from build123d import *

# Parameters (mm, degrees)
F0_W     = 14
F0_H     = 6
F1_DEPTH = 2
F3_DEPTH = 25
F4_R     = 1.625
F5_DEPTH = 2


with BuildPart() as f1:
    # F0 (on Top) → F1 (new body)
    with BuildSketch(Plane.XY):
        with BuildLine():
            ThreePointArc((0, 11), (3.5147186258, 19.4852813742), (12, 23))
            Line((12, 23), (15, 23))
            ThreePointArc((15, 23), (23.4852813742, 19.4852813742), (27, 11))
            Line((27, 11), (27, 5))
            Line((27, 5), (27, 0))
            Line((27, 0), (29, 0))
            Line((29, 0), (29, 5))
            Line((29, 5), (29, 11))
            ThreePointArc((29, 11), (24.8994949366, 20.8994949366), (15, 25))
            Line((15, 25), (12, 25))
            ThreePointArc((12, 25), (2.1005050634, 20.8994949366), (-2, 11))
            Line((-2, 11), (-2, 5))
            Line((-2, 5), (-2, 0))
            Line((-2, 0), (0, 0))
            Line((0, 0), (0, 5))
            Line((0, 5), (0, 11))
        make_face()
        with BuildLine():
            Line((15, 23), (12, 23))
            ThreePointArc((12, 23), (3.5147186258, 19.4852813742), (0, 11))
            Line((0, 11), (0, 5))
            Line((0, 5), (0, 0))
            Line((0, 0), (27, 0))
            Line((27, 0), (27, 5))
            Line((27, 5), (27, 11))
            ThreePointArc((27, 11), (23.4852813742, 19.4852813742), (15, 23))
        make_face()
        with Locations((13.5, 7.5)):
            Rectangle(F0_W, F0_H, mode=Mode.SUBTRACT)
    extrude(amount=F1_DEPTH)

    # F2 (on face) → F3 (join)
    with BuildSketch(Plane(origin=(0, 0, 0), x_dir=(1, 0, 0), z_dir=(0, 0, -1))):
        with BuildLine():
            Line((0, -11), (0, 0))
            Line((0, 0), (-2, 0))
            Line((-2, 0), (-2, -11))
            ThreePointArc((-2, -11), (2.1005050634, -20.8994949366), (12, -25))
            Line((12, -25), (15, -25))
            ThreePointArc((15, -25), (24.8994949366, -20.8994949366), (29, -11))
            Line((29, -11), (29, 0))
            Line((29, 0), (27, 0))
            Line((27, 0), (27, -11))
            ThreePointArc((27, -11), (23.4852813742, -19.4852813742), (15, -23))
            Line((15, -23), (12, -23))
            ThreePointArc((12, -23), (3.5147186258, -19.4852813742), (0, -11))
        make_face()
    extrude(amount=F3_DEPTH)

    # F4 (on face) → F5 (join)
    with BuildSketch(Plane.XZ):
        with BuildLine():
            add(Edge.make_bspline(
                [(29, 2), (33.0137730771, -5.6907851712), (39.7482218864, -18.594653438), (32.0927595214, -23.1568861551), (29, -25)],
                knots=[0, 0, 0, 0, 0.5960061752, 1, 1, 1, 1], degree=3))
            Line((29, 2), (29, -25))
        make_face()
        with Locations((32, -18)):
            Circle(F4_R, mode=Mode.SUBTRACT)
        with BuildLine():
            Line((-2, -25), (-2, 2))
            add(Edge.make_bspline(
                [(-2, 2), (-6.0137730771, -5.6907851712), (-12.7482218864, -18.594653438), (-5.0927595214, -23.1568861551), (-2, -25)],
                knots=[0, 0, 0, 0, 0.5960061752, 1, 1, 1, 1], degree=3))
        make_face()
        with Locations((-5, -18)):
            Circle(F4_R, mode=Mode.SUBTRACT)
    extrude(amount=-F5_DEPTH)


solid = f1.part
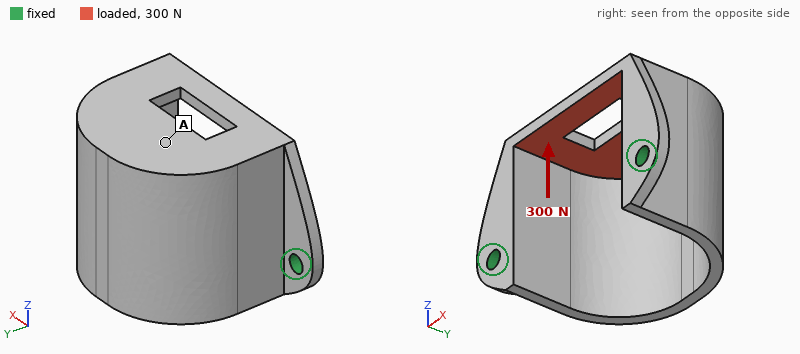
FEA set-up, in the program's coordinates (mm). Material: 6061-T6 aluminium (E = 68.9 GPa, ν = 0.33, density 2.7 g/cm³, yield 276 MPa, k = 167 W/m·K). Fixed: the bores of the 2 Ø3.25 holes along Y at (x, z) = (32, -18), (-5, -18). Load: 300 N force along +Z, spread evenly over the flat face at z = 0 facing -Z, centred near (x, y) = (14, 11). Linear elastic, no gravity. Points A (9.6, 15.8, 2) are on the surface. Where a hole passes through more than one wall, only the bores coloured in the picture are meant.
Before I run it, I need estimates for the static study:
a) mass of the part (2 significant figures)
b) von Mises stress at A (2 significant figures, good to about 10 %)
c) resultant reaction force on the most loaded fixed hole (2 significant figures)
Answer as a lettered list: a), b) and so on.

a) 13 g
b) 15 MPa
c) 150 N
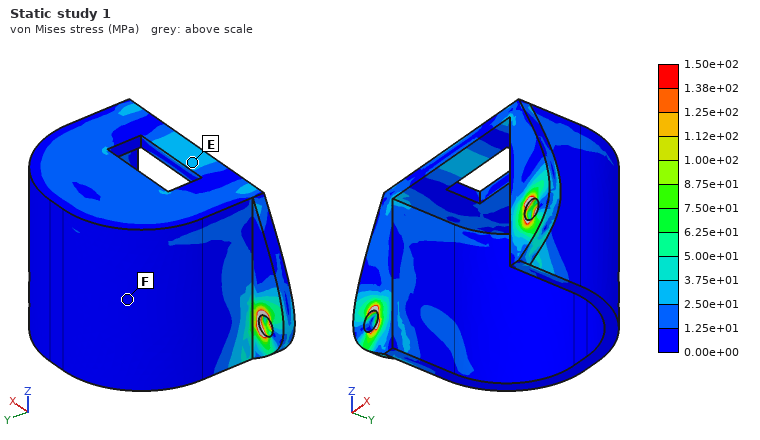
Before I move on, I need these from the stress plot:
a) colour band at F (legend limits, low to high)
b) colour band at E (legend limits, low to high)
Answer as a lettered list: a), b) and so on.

a) 0.00e+00 to 1.25e+01 MPa
b) 2.50e+01 to 3.75e+01 MPa
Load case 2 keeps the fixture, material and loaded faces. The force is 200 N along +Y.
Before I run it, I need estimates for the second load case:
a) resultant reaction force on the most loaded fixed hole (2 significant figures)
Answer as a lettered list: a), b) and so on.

a) 100 N
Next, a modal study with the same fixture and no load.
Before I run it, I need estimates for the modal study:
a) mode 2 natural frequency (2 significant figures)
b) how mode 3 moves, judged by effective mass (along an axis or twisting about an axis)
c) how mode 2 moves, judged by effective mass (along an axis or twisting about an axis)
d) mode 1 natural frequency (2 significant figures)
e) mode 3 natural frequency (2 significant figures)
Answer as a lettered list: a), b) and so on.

a) 3500 Hz
b) along X
c) along X
d) 2000 Hz
e) 6600 Hz
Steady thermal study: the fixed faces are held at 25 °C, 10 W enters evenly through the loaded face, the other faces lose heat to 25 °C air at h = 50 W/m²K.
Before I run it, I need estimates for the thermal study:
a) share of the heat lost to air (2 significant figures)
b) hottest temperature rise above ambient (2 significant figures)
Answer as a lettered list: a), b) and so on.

a) 22 %
b) 17 K
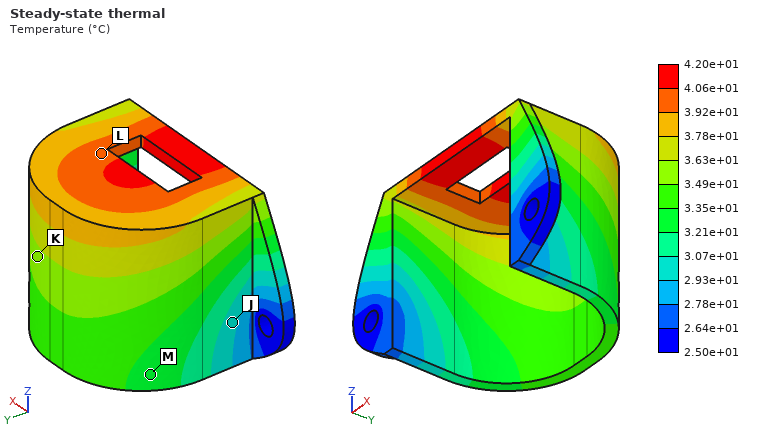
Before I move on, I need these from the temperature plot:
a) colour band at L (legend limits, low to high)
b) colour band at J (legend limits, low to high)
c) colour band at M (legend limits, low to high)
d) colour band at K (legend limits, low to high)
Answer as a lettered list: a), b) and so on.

a) 3.92e+01 to 4.06e+01 °C
b) 2.93e+01 to 3.07e+01 °C
c) 3.21e+01 to 3.35e+01 °C
d) 3.49e+01 to 3.63e+01 °C
